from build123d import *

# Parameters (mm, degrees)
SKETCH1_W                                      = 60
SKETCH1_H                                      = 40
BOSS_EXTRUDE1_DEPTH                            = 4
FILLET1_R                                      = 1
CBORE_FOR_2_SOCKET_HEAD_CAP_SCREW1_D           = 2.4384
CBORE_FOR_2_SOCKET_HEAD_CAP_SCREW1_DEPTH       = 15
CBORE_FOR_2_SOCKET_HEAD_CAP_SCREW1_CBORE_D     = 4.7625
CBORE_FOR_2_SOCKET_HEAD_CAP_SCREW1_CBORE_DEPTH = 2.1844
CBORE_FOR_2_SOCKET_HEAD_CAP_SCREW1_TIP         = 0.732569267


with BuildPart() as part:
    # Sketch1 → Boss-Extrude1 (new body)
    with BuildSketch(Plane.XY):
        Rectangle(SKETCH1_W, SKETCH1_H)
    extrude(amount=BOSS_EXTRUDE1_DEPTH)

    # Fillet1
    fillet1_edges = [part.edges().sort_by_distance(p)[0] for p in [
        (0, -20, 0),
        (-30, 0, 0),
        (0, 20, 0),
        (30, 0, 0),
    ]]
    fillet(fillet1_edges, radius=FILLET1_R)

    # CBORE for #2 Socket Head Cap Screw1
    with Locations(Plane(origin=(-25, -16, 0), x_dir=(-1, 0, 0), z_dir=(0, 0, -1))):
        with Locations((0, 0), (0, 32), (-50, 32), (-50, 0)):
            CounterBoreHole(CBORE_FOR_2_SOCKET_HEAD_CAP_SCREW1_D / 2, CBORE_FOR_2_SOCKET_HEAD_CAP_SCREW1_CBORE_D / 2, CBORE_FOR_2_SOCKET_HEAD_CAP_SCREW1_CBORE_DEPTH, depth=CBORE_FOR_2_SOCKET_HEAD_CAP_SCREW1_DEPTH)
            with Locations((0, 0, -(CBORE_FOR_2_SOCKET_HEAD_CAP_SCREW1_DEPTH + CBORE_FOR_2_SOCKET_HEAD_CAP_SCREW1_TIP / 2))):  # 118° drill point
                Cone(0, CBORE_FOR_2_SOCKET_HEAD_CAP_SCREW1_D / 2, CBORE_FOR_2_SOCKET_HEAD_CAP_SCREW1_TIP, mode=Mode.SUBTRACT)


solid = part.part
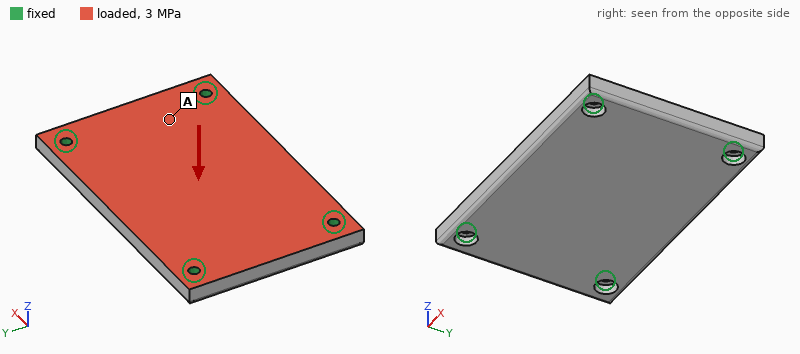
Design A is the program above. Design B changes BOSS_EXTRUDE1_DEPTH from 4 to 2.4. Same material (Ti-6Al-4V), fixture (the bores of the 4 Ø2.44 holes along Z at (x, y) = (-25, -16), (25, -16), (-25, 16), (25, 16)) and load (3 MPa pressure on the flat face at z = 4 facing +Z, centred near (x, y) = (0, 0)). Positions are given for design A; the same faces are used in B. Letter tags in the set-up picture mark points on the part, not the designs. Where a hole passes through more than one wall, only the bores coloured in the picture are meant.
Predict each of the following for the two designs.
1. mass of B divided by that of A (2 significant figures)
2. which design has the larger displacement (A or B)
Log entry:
0.59
B
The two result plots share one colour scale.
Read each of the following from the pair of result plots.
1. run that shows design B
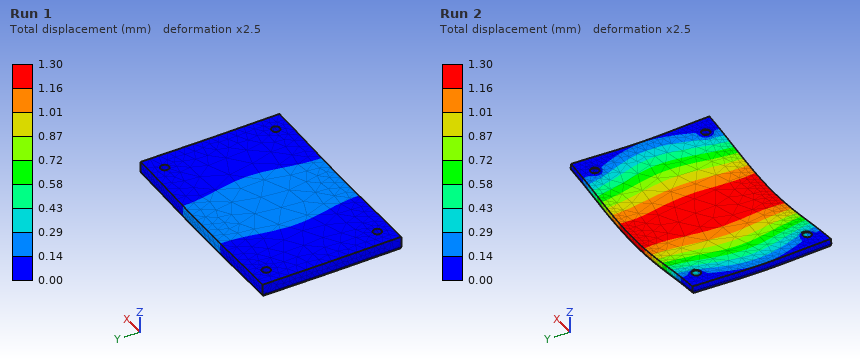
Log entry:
Run 2
